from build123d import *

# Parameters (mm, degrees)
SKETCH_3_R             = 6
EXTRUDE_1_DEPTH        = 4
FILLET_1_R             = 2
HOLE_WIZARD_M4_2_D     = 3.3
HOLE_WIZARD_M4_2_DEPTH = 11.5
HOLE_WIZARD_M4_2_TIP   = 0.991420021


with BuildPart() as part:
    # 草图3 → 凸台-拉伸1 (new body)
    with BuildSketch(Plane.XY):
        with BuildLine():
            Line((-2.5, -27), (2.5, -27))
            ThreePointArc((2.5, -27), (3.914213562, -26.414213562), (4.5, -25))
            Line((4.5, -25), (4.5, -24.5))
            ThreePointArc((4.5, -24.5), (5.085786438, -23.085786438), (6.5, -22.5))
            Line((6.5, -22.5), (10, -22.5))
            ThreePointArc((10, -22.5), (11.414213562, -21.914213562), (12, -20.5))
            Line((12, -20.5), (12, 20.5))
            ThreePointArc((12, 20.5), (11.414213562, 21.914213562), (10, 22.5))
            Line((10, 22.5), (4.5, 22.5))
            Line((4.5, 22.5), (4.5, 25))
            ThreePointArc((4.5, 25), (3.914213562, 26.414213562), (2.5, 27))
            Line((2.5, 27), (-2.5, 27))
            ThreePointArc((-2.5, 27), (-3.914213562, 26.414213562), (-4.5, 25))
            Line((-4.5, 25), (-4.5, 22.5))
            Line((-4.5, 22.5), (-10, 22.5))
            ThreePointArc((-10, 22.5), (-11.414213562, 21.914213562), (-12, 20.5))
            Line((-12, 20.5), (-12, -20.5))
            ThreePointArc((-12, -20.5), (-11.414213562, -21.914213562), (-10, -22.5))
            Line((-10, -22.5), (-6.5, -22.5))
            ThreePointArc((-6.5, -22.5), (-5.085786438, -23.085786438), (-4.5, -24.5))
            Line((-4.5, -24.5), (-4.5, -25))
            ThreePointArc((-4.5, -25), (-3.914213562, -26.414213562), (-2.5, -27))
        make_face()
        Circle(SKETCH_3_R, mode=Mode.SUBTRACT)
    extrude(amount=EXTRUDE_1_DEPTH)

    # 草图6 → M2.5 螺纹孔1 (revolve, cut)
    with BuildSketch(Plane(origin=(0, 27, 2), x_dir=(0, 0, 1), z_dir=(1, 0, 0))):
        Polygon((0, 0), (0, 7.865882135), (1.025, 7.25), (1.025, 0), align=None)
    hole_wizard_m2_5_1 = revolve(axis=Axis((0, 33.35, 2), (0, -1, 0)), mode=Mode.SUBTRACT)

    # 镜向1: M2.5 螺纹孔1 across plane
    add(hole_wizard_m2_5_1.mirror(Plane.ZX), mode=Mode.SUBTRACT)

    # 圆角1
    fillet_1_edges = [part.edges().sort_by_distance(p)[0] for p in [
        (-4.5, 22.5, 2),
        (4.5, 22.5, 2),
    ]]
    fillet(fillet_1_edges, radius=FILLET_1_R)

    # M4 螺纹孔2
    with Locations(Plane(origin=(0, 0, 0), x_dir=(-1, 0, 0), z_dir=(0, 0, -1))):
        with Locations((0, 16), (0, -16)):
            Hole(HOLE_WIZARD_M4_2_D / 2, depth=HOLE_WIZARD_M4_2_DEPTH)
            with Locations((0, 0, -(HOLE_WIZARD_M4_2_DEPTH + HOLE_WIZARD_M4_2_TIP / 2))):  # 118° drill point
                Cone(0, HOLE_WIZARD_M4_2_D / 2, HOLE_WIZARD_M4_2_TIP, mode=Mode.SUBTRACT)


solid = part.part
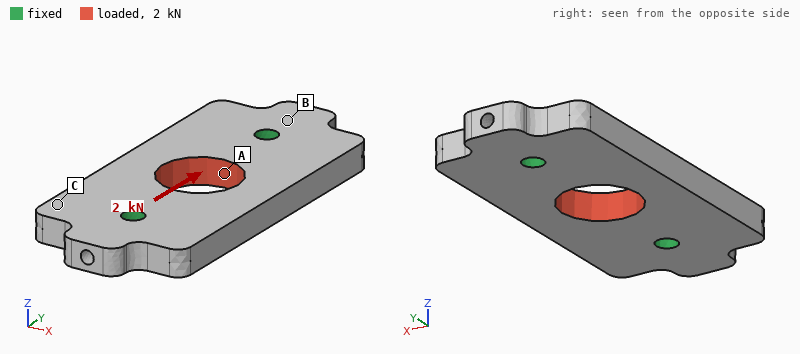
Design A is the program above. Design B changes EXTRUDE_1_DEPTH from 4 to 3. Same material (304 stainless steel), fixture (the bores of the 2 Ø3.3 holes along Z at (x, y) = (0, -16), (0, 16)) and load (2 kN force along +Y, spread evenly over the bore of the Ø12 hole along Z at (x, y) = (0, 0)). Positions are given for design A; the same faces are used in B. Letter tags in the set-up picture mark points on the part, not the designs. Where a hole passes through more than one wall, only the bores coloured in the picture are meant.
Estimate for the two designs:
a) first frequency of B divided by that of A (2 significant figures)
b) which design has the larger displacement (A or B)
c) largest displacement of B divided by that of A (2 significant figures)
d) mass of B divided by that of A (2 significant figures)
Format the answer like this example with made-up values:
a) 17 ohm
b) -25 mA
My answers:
a) 0.80
b) B
c) 1.4
d) 0.75
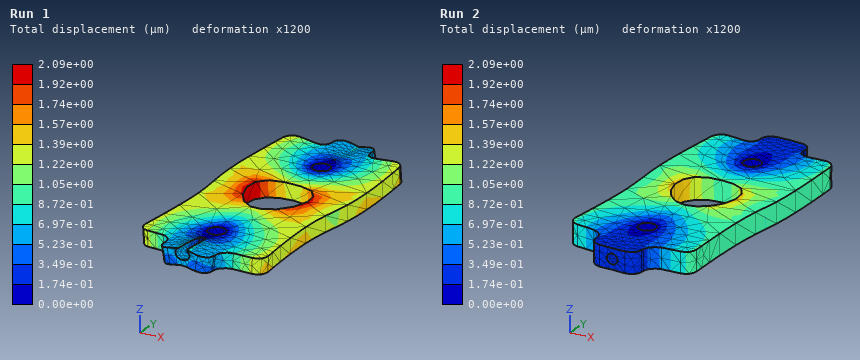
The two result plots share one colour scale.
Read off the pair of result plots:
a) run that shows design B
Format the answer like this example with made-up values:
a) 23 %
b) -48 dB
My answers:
a) Run 1
